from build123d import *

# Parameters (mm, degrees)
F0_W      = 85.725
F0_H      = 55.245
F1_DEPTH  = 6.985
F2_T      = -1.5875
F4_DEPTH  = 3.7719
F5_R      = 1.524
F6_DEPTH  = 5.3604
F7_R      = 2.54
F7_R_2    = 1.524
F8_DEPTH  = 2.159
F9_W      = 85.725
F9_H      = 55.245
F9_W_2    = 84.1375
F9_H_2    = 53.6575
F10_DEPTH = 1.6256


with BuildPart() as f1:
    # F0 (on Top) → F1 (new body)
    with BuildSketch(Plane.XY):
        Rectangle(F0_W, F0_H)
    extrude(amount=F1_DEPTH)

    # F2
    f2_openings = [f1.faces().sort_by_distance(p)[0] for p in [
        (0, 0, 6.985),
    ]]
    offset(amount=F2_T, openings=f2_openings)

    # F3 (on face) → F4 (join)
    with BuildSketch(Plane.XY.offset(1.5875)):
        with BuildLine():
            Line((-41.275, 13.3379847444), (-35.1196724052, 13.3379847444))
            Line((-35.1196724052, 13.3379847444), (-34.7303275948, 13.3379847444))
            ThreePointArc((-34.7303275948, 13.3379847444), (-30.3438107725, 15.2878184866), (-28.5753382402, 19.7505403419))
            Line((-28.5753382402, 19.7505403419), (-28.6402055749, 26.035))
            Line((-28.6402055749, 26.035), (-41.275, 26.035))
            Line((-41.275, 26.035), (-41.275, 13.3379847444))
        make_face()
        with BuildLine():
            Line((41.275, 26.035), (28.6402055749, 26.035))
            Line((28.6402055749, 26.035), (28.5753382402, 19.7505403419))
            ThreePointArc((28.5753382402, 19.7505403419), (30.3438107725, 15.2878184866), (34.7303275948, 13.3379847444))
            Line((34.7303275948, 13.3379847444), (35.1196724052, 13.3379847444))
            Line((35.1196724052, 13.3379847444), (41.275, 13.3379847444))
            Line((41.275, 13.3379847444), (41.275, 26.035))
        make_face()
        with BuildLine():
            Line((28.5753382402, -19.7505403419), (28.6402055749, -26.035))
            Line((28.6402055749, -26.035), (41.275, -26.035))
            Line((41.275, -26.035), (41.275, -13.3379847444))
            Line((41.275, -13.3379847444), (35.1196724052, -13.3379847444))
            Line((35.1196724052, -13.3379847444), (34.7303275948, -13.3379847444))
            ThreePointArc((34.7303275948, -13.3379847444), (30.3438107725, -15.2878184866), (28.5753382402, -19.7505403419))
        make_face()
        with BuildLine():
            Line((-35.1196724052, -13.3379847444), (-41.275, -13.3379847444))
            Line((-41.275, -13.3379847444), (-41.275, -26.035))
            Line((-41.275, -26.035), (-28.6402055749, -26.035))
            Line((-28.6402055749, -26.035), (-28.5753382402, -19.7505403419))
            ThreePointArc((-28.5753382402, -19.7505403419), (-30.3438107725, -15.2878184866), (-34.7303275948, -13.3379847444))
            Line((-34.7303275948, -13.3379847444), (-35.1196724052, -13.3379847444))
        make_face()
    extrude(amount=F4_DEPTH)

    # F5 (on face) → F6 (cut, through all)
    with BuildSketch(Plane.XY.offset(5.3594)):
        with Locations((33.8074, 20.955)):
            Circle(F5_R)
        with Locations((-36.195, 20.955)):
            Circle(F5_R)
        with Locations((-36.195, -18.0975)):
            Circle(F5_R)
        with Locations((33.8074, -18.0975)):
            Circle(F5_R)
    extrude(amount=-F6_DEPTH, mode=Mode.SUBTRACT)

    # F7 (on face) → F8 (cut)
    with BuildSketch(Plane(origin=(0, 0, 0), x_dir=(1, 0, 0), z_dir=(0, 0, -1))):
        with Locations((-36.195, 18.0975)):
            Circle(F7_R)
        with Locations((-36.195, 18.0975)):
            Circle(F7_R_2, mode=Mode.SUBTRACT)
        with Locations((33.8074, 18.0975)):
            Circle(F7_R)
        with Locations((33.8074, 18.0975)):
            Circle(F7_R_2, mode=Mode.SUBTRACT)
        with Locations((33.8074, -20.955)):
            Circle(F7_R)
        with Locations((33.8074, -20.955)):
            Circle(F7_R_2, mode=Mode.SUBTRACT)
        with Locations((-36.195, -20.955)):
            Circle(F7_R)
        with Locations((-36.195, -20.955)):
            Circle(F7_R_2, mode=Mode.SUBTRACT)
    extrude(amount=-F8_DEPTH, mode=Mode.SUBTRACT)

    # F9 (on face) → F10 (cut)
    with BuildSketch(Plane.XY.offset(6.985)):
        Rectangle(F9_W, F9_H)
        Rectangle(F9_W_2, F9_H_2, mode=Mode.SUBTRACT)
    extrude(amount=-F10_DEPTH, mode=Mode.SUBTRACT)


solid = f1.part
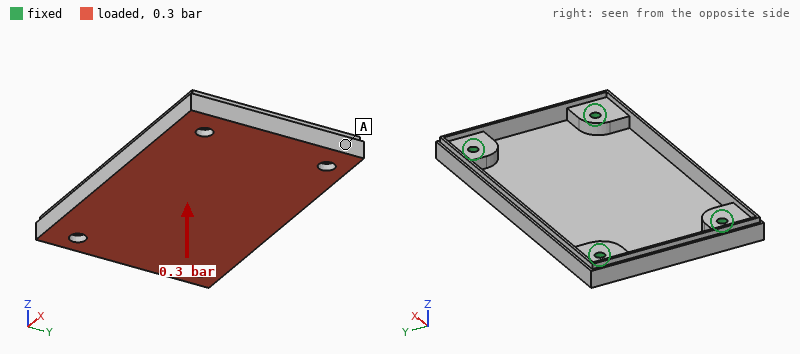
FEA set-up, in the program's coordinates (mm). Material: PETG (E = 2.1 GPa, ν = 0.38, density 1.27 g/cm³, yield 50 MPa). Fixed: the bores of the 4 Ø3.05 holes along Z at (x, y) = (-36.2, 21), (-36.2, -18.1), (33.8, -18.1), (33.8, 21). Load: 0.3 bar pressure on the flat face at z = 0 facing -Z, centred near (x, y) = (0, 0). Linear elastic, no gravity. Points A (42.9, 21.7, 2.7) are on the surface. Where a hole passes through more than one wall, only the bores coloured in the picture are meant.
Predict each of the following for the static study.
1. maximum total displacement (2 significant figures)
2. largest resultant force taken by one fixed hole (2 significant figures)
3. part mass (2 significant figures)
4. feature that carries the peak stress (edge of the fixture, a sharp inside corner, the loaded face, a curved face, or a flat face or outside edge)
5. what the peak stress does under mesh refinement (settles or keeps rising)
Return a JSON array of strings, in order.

["1.2 mm", "53 N", "15 g", "edge of the fixture", "keeps rising"]
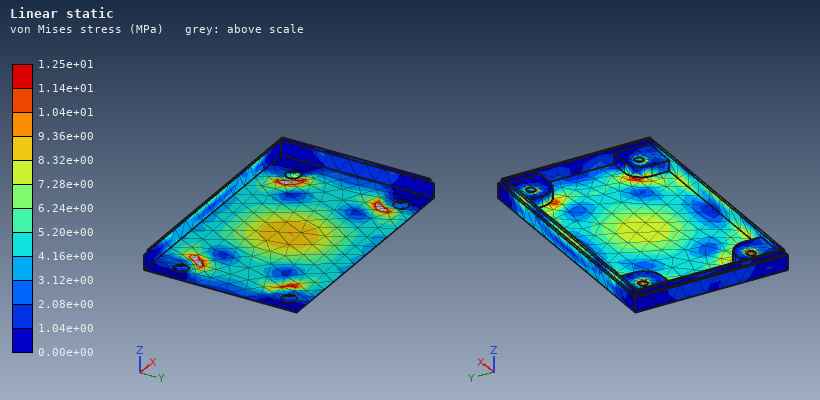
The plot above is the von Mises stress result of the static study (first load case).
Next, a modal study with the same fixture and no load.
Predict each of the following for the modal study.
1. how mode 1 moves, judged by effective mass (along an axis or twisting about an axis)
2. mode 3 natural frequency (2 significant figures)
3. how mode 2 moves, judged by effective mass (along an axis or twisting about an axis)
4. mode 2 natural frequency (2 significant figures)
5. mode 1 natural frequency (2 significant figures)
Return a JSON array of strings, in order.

["along Z", "1500 Hz", "twisting about X", "1300 Hz", "700 Hz"]
